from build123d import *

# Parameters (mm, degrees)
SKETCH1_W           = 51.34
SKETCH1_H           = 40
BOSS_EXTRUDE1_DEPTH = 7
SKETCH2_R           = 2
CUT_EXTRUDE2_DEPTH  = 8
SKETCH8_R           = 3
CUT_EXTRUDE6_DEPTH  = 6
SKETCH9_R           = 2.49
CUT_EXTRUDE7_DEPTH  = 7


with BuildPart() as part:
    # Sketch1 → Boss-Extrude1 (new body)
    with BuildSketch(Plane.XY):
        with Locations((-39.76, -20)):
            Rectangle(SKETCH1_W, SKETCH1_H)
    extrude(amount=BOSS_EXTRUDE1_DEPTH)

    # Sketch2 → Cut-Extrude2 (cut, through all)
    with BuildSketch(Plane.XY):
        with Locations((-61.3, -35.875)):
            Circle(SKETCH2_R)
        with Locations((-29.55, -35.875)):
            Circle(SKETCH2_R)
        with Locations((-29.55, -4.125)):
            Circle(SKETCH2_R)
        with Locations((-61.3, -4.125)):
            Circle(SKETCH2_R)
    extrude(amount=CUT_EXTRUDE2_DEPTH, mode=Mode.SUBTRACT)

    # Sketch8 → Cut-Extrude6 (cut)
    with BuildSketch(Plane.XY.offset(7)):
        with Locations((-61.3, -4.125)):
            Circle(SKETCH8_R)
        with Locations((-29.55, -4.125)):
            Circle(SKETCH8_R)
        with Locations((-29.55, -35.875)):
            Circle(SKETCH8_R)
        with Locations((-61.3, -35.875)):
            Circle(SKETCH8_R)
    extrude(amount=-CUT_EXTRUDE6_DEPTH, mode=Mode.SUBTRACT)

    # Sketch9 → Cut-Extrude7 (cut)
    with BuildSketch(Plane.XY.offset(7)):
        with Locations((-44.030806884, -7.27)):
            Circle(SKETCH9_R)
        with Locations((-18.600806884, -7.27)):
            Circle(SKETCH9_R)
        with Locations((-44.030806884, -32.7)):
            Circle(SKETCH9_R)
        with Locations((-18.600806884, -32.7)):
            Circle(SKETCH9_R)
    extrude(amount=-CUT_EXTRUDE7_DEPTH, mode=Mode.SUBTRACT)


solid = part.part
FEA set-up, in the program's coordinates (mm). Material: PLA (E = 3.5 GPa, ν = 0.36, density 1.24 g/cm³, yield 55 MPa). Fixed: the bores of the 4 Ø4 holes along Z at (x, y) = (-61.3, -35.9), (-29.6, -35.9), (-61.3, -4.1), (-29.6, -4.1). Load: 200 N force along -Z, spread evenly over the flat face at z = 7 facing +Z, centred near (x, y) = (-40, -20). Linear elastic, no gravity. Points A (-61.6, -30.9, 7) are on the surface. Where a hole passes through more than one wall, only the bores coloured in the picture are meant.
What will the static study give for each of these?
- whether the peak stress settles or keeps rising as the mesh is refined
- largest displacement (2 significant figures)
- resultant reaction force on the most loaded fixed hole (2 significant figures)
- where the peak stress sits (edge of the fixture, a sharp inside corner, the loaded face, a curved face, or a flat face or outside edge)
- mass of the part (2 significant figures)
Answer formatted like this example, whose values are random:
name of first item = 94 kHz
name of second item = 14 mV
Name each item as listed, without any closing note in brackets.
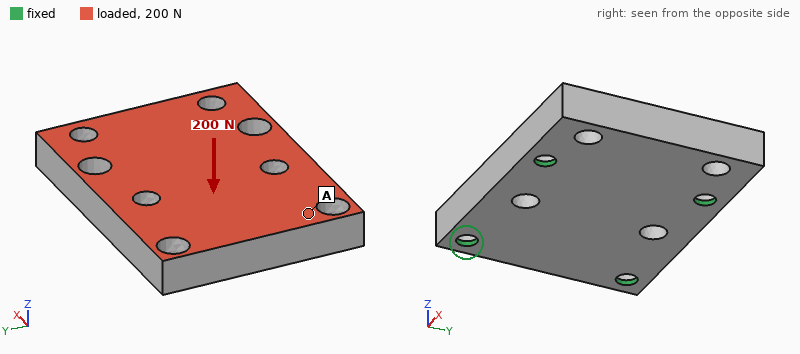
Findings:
whether the peak stress settles or keeps rising as the mesh is refined = keeps rising
largest displacement = 35 µm
resultant reaction force on the most loaded fixed hole = 76 N
where the peak stress sits = edge of the fixture
mass of the part = 16 g
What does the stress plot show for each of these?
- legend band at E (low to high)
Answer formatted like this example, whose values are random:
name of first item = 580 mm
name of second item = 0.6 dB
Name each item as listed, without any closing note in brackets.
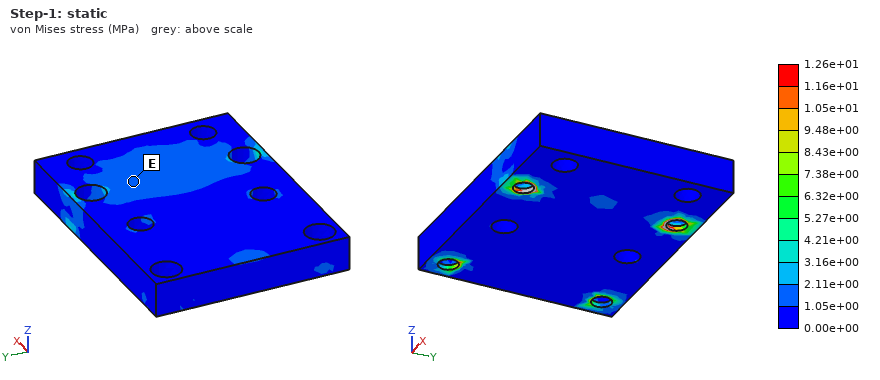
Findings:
legend band at E = 1.05e+00 to 2.11e+00 MPa
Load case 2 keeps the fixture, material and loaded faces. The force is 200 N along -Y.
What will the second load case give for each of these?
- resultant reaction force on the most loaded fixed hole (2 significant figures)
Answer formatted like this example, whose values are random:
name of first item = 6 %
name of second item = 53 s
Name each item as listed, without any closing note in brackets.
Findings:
resultant reaction force on the most loaded fixed hole = 64 N
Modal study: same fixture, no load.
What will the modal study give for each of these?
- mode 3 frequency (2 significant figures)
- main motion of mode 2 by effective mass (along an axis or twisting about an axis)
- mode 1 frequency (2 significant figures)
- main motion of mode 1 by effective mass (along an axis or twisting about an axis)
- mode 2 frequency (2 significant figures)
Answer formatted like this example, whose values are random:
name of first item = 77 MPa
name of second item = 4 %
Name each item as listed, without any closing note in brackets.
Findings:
mode 3 frequency = 6200 Hz
main motion of mode 2 by effective mass = along Z
mode 1 frequency = 3500 Hz
main motion of mode 1 by effective mass = along Z
mode 2 frequency = 4700 Hz
